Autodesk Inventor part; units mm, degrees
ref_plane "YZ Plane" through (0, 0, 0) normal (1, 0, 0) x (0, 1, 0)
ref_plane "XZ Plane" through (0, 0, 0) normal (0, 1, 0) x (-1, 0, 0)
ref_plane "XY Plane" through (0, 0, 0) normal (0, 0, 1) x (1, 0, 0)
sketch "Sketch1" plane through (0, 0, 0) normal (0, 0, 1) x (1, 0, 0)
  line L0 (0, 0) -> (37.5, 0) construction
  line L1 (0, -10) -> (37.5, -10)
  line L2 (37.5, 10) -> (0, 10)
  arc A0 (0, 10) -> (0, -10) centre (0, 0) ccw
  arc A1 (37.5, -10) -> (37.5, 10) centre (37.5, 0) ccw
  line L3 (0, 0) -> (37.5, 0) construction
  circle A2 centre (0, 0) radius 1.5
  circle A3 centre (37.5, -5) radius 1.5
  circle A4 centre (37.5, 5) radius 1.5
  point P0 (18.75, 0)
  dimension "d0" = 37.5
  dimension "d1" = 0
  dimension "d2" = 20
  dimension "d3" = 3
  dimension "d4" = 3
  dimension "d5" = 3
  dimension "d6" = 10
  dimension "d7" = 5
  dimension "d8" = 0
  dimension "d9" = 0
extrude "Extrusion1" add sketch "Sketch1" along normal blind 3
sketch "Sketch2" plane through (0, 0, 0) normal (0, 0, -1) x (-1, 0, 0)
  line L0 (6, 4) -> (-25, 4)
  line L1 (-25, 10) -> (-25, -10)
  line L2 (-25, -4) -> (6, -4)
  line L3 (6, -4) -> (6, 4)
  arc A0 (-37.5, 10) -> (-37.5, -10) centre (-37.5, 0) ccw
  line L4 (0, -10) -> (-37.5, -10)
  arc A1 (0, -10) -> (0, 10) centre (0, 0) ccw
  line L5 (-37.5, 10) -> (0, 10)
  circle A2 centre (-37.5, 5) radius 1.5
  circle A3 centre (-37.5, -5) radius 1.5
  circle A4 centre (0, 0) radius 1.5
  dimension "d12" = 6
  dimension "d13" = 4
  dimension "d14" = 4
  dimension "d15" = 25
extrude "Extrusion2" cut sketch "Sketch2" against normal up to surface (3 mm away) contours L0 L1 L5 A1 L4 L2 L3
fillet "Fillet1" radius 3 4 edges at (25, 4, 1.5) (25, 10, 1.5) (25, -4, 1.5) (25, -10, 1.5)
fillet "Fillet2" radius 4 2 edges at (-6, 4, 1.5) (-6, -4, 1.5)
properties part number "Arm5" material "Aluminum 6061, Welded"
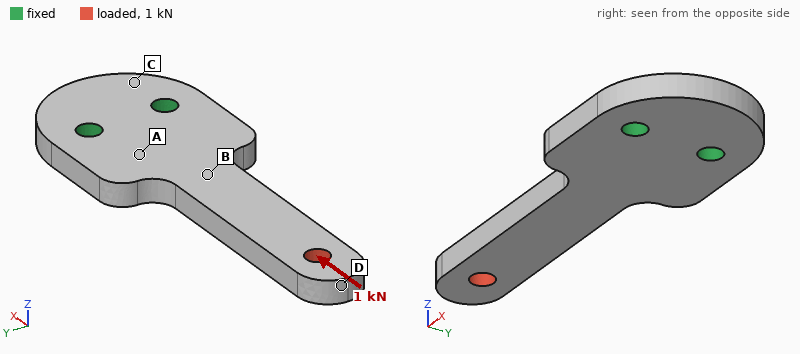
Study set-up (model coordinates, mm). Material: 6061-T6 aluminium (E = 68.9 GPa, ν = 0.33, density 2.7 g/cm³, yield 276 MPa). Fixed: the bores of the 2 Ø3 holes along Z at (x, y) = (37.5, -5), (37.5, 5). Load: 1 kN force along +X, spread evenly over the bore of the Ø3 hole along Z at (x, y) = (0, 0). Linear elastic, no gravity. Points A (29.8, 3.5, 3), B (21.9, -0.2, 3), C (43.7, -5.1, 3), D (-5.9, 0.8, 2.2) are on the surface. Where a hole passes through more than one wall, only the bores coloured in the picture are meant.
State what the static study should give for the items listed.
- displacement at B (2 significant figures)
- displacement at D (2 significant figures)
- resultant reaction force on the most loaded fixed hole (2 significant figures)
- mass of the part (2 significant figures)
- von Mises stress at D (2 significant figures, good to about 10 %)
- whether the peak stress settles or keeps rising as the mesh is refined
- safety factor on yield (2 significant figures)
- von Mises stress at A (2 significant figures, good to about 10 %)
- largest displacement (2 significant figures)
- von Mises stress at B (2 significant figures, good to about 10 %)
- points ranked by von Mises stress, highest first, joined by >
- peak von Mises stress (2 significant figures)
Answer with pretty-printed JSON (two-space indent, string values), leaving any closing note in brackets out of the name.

{
  "displacement at B": "6.2 µm",
  "displacement at D": "21 µm",
  "resultant reaction force on the most loaded fixed hole": "510 N",
  "mass of the part": "5.1 g",
  "von Mises stress at D": "12 MPa",
  "whether the peak stress settles or keeps rising as the mesh is refined": "settles",
  "safety factor on yield": "2.7",
  "von Mises stress at A": "26 MPa",
  "largest displacement": "22 µm",
  "von Mises stress at B": "34 MPa",
  "points ranked by von Mises stress, highest first, joined by >": "B > A > D > C",
  "peak von Mises stress": "100 MPa"
}
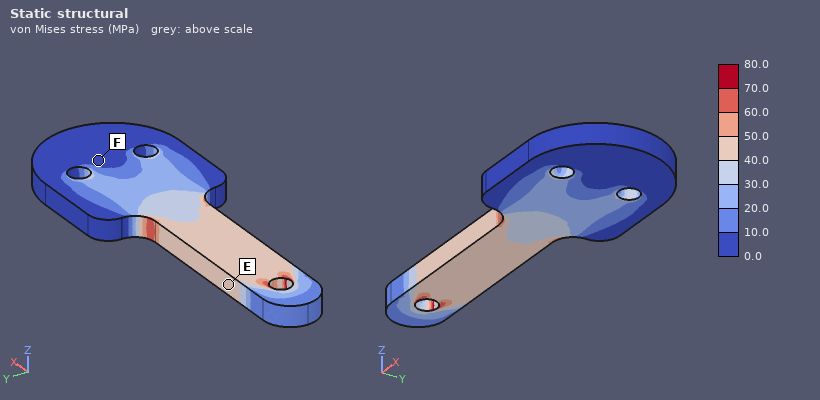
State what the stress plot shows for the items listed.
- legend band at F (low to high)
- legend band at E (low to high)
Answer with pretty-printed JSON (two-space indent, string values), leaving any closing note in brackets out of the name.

{
  "legend band at F": "0.0 to 10.0 MPa",
  "legend band at E": "40.0 to 50.0 MPa"
}
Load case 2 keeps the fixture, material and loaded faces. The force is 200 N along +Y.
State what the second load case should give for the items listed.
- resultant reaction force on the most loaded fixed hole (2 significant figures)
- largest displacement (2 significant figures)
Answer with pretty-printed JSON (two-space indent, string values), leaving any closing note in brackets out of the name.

{
  "resultant reaction force on the most loaded fixed hole": "640 N",
  "largest displacement": "0.21 mm"
}
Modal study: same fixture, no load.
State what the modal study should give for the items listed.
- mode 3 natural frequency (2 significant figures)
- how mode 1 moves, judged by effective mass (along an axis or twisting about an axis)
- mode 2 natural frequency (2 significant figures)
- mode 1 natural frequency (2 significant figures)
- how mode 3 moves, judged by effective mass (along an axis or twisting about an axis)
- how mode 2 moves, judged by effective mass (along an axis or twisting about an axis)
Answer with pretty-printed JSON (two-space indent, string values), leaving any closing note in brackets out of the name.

{
  "mode 3 natural frequency": "9400 Hz",
  "how mode 1 moves, judged by effective mass": "along Z",
  "mode 2 natural frequency": "6200 Hz",
  "mode 1 natural frequency": "1800 Hz",
  "how mode 3 moves, judged by effective mass": "along Z",
  "how mode 2 moves, judged by effective mass": "along Y"
}
